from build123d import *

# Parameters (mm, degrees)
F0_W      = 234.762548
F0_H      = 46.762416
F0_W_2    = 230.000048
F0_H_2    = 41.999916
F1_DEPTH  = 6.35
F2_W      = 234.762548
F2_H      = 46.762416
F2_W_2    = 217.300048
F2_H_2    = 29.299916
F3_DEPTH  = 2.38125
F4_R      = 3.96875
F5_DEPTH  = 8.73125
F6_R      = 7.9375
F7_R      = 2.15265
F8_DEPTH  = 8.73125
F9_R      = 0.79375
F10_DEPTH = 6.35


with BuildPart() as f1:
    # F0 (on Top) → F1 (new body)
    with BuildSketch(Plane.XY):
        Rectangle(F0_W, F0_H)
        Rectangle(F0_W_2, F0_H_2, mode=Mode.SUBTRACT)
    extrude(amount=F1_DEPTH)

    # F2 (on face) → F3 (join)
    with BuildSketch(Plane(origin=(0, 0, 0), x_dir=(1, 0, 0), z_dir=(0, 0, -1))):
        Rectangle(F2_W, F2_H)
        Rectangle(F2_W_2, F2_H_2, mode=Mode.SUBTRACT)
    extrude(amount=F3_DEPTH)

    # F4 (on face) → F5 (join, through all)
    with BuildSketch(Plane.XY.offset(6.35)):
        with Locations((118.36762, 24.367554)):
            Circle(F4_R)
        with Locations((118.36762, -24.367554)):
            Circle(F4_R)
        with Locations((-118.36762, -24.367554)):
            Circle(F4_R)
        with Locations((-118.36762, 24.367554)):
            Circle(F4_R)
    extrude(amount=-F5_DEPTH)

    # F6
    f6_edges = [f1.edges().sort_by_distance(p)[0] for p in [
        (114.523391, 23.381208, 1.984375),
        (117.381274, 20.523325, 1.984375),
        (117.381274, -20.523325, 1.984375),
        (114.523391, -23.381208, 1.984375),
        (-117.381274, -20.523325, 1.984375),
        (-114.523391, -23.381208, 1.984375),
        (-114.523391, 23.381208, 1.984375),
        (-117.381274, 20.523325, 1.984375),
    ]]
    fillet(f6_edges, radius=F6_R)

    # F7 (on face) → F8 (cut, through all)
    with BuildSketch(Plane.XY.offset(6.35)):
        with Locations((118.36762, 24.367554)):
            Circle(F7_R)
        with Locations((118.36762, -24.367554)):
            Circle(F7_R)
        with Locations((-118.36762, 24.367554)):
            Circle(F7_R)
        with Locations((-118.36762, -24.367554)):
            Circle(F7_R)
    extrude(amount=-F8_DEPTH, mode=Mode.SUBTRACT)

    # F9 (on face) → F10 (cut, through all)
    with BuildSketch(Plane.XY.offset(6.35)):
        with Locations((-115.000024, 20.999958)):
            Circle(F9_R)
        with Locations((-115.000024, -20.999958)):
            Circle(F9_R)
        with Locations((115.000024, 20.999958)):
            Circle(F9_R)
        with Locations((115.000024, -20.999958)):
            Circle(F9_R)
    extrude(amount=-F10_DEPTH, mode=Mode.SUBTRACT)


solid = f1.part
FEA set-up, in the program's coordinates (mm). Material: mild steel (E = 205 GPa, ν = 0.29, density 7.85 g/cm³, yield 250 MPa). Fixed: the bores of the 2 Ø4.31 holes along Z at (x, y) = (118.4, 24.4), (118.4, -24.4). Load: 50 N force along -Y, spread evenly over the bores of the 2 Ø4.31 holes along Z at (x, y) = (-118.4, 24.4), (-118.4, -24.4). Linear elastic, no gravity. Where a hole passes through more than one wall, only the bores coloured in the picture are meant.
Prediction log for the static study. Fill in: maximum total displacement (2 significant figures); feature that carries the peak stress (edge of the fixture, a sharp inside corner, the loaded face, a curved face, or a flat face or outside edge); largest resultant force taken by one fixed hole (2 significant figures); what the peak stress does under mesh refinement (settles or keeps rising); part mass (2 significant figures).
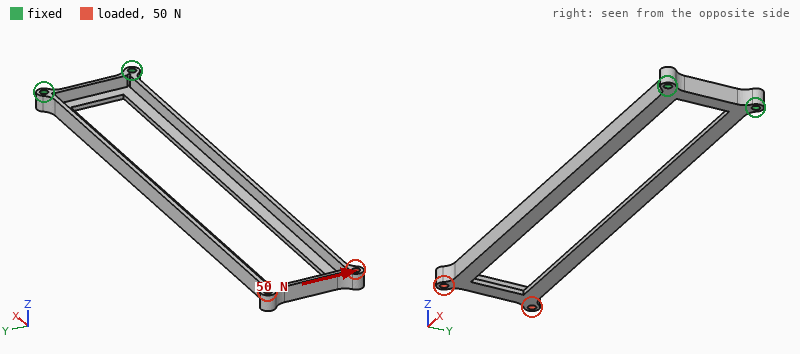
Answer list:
0.79 mm
a sharp inside corner
210 N
keeps rising
160 g
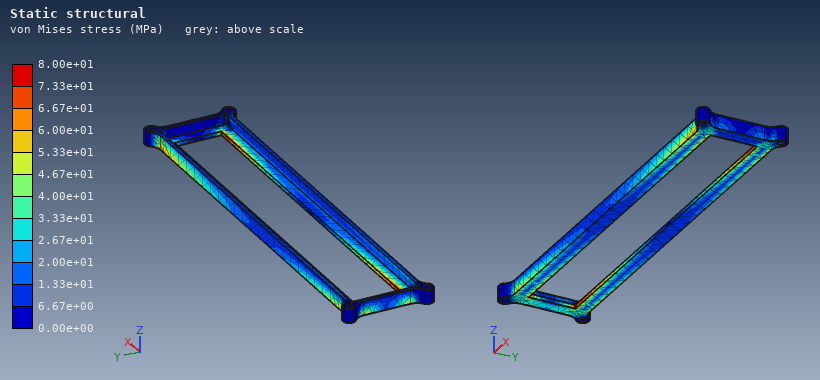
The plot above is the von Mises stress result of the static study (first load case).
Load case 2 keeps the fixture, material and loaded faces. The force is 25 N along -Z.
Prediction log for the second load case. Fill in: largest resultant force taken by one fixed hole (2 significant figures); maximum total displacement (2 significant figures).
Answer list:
110 N
1.2 mm
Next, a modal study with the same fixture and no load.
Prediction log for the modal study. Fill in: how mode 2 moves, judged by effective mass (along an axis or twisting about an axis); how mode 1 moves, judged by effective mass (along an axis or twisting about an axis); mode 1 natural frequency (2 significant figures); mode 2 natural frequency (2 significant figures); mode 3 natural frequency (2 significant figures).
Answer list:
along Y
along Z
110 Hz
160 Hz
290 Hz
